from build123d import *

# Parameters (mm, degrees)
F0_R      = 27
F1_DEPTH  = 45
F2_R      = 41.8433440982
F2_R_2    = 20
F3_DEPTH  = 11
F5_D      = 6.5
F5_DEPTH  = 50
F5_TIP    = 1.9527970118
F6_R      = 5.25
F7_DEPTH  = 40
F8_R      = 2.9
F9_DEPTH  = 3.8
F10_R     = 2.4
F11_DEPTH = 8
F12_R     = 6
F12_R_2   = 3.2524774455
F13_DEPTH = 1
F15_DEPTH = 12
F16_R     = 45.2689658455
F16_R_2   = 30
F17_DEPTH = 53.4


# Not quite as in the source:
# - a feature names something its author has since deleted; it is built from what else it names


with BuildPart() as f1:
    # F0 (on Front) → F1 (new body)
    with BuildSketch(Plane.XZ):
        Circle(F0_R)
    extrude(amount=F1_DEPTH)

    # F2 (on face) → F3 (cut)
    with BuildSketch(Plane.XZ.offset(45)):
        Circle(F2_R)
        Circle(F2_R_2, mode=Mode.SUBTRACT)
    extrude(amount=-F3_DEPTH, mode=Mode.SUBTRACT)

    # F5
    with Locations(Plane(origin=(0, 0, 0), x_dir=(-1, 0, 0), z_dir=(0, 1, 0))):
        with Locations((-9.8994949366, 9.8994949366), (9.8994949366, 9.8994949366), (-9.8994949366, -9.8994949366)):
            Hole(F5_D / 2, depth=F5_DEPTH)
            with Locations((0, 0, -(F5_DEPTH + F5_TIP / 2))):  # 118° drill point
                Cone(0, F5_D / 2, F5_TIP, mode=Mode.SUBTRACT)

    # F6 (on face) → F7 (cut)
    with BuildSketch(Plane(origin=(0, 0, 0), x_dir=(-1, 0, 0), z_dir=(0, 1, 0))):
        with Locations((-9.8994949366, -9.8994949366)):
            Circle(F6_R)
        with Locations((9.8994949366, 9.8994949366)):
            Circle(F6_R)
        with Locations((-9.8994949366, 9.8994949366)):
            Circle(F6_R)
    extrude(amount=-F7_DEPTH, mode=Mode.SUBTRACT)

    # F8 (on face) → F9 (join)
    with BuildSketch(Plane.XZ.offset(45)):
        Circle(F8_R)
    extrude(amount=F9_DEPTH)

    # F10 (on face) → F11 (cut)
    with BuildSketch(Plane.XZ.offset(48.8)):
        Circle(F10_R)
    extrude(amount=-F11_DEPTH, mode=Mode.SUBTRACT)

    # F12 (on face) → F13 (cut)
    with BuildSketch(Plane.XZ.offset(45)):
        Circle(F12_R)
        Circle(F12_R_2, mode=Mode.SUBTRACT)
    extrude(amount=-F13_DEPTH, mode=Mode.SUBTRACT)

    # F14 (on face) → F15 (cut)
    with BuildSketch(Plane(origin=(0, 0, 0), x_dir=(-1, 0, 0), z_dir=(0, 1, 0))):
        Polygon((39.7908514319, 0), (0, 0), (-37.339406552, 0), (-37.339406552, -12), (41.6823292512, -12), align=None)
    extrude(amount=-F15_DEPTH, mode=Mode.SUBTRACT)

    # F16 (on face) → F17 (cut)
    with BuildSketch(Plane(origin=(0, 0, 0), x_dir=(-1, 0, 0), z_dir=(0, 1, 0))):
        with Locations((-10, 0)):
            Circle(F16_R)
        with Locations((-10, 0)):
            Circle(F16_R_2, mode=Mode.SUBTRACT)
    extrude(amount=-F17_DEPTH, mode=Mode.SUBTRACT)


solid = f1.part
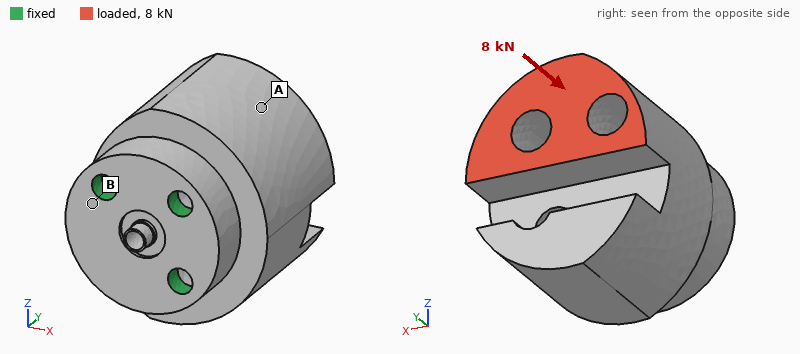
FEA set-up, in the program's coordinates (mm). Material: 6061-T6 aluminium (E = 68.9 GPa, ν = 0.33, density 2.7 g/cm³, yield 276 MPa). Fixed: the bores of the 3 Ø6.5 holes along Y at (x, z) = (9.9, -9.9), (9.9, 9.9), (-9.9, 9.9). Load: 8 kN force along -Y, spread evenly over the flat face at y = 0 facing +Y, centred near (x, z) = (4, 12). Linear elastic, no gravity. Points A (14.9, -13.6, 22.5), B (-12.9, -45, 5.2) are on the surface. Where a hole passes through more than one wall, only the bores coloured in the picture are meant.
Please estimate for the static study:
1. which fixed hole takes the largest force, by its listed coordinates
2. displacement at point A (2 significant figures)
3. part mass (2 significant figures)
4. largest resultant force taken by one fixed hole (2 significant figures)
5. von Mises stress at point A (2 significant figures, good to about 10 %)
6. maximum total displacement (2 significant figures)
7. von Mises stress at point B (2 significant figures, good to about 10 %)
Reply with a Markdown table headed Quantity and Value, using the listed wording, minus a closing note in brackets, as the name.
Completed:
| Quantity | Value |
|---|---|
| which fixed hole takes the largest force, by its listed coordinates | (9.9, 9.9) |
| displacement at point A | 31 µm |
| part mass | 170 g |
| largest resultant force taken by one fixed hole | 5.2 kN |
| von Mises stress at point A | 10 MPa |
| maximum total displacement | 40 µm |
| von Mises stress at point B | 18 MPa |
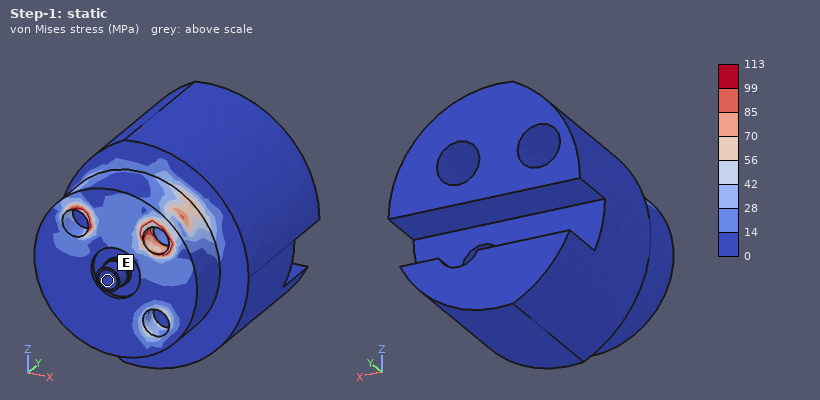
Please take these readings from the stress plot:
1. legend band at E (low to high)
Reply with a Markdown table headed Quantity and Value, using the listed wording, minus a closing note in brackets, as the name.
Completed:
| Quantity | Value |
|---|---|
| legend band at E | 0 to 14 MPa |
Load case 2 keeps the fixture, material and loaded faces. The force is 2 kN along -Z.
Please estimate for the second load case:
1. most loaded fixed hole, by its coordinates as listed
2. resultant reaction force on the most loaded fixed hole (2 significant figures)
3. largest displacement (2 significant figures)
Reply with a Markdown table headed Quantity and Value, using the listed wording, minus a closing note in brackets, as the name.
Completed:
| Quantity | Value |
|---|---|
| most loaded fixed hole, by its coordinates as listed | (9.9, -9.9) |
| resultant reaction force on the most loaded fixed hole | 3.5 kN |
| largest displacement | 45 µm |
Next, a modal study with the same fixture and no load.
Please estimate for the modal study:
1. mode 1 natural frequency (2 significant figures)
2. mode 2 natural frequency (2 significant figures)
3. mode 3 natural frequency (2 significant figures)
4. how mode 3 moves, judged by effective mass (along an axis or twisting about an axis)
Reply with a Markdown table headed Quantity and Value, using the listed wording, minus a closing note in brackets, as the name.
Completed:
| Quantity | Value |
|---|---|
| mode 1 natural frequency | 4000 Hz |
| mode 2 natural frequency | 6000 Hz |
| mode 3 natural frequency | 10 kHz |
| how mode 3 moves, judged by effective mass | twisting about Y |
